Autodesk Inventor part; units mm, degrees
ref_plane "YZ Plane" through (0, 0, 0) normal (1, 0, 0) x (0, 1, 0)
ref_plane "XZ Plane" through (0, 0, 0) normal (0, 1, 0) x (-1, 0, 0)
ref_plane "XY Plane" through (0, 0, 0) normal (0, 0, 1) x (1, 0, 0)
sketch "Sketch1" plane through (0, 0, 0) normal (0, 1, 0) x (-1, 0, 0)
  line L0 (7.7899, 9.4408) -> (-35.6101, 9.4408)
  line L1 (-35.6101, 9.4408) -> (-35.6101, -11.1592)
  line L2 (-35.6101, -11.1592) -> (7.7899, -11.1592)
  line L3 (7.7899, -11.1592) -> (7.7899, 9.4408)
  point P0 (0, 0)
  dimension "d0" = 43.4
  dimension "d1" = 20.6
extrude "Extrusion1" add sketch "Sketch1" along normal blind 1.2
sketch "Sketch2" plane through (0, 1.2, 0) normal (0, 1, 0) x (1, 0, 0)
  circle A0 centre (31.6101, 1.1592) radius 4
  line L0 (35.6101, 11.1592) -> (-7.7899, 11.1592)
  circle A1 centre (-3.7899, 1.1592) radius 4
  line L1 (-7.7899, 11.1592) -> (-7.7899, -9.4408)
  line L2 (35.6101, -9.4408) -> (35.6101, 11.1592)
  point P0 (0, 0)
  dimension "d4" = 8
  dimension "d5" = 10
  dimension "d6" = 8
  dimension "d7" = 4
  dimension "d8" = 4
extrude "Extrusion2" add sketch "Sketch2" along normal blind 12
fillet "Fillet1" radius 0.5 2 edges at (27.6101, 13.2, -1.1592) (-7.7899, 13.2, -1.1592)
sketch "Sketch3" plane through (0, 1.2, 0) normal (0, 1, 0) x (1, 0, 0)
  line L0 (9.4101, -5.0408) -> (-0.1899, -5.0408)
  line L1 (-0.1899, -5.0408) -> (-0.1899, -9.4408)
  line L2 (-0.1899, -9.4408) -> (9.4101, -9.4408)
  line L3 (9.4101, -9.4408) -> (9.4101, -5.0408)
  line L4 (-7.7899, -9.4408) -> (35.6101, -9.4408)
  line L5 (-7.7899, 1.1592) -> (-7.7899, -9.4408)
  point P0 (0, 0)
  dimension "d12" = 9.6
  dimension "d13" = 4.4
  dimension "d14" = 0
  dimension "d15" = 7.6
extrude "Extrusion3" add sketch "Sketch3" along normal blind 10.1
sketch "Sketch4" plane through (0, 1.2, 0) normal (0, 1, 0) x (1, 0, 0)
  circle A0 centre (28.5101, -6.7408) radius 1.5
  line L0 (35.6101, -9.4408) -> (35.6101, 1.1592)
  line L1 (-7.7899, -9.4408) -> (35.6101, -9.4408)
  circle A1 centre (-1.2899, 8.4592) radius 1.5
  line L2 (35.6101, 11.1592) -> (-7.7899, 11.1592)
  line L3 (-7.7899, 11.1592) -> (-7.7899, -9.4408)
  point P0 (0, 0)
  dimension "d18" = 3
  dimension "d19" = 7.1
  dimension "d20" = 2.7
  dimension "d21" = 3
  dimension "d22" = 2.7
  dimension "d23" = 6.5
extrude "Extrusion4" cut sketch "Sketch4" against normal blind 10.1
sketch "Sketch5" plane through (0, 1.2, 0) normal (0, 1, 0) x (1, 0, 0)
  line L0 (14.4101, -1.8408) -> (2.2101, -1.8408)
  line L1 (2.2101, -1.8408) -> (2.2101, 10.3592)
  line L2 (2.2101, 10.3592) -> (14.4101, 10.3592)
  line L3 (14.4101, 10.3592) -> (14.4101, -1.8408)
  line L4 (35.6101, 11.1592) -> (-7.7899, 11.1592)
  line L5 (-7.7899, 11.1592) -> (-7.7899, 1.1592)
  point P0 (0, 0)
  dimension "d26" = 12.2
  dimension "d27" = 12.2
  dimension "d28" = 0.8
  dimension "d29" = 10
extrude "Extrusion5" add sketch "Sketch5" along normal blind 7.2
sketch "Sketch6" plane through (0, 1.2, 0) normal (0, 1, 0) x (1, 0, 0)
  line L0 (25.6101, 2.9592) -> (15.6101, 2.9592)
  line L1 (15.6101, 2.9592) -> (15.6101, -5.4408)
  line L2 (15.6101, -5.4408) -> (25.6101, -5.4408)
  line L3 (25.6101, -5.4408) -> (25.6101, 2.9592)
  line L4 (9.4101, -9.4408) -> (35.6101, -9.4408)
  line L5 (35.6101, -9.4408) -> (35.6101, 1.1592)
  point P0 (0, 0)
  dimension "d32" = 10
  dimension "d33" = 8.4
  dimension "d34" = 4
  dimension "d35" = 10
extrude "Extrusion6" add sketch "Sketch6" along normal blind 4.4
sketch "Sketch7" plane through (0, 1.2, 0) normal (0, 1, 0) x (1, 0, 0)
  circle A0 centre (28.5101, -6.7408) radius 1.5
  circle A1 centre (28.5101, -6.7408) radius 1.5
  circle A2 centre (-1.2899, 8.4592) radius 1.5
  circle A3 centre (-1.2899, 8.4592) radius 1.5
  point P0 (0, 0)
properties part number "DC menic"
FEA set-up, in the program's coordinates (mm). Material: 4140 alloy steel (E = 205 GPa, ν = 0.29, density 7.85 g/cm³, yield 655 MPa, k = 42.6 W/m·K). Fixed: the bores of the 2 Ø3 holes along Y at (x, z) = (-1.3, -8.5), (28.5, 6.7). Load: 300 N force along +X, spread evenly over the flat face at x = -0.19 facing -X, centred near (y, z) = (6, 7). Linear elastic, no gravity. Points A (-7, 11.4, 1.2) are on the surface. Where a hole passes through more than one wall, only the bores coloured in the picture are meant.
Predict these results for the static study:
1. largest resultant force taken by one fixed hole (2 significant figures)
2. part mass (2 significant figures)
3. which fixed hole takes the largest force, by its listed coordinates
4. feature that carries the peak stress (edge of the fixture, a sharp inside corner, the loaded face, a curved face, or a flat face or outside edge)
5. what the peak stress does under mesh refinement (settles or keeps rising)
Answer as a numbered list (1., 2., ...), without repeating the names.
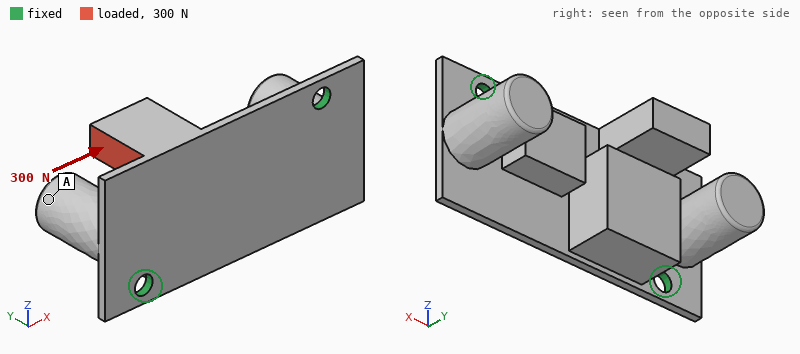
1. 190 N
2. 32 g
3. (28.5, 6.7)
4. edge of the fixture
5. keeps rising
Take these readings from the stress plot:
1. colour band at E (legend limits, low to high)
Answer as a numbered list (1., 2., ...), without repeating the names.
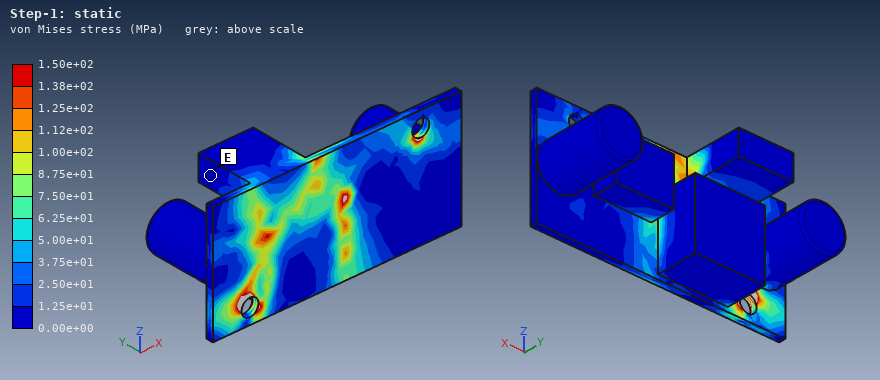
1. 0.00e+00 to 1.25e+01 MPa
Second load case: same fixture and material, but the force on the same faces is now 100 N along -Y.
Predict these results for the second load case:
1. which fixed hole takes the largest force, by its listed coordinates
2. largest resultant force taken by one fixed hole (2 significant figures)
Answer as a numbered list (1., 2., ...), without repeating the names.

1. (-1.3, -8.5)
2. 89 N
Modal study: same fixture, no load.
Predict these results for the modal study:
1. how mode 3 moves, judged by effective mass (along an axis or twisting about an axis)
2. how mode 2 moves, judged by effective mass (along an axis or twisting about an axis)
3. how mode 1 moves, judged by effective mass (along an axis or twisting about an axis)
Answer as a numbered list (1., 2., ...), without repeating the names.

1. along Y
2. along Y
3. along Z
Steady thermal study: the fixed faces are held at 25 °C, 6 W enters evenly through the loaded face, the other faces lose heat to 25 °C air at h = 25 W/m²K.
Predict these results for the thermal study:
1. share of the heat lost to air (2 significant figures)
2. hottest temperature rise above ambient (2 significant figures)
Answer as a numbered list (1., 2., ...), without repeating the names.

1. 28 %
2. 78 K
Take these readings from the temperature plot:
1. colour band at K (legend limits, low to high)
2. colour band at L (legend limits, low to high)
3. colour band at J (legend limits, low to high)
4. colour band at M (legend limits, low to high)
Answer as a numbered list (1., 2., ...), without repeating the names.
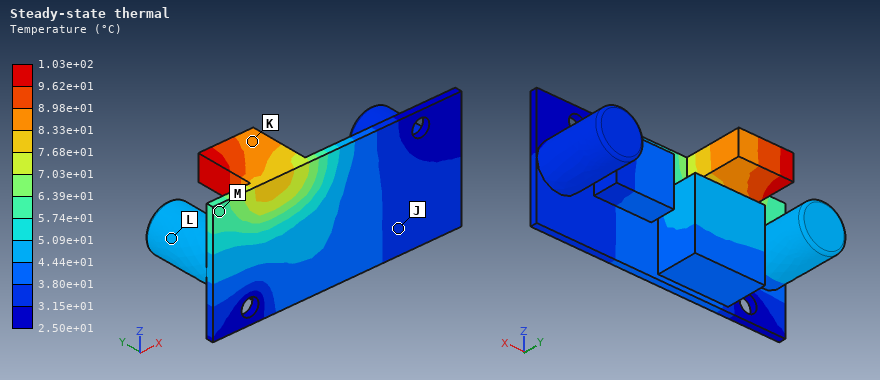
1. 8.33e+01 to 8.98e+01 °C
2. 4.44e+01 to 5.09e+01 °C
3. 3.15e+01 to 3.80e+01 °C
4. 5.74e+01 to 6.39e+01 °C
